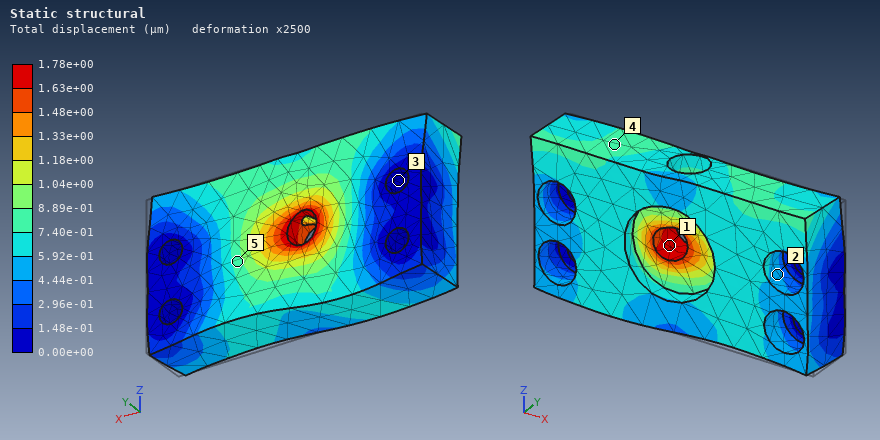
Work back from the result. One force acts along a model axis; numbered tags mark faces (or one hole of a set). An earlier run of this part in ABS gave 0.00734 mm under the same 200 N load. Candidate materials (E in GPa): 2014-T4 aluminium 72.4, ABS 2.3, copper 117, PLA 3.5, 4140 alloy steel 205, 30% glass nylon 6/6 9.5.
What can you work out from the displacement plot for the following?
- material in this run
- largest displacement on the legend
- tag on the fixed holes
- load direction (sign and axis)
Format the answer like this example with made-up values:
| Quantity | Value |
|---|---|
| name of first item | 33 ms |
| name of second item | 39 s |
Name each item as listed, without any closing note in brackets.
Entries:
| Quantity | Value |
|---|---|
| material in this run | 30% glass nylon 6/6 |
| largest displacement on the legend | 1.78e+00 µm |
| tag on the fixed holes | 3 |
| load direction | -X |
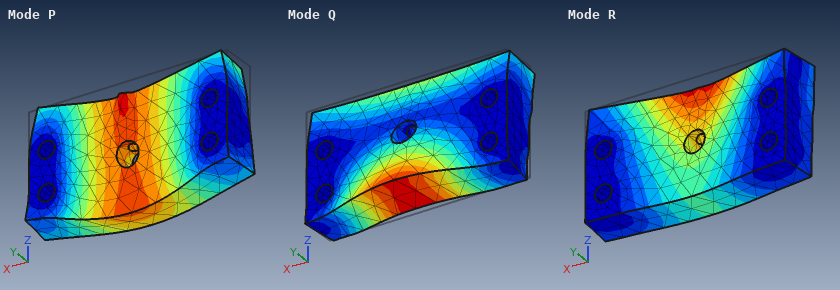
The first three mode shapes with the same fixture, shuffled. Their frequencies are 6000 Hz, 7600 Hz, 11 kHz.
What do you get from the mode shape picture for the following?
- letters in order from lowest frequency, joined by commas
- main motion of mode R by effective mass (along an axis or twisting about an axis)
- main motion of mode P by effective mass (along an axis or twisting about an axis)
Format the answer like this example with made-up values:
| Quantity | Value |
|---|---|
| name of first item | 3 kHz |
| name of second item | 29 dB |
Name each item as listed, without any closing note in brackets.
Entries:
| Quantity | Value |
|---|---|
| letters in order from lowest frequency, joined by commas | R, Q, P |
| main motion of mode R by effective mass | along Y |
| main motion of mode P by effective mass | along Z |
